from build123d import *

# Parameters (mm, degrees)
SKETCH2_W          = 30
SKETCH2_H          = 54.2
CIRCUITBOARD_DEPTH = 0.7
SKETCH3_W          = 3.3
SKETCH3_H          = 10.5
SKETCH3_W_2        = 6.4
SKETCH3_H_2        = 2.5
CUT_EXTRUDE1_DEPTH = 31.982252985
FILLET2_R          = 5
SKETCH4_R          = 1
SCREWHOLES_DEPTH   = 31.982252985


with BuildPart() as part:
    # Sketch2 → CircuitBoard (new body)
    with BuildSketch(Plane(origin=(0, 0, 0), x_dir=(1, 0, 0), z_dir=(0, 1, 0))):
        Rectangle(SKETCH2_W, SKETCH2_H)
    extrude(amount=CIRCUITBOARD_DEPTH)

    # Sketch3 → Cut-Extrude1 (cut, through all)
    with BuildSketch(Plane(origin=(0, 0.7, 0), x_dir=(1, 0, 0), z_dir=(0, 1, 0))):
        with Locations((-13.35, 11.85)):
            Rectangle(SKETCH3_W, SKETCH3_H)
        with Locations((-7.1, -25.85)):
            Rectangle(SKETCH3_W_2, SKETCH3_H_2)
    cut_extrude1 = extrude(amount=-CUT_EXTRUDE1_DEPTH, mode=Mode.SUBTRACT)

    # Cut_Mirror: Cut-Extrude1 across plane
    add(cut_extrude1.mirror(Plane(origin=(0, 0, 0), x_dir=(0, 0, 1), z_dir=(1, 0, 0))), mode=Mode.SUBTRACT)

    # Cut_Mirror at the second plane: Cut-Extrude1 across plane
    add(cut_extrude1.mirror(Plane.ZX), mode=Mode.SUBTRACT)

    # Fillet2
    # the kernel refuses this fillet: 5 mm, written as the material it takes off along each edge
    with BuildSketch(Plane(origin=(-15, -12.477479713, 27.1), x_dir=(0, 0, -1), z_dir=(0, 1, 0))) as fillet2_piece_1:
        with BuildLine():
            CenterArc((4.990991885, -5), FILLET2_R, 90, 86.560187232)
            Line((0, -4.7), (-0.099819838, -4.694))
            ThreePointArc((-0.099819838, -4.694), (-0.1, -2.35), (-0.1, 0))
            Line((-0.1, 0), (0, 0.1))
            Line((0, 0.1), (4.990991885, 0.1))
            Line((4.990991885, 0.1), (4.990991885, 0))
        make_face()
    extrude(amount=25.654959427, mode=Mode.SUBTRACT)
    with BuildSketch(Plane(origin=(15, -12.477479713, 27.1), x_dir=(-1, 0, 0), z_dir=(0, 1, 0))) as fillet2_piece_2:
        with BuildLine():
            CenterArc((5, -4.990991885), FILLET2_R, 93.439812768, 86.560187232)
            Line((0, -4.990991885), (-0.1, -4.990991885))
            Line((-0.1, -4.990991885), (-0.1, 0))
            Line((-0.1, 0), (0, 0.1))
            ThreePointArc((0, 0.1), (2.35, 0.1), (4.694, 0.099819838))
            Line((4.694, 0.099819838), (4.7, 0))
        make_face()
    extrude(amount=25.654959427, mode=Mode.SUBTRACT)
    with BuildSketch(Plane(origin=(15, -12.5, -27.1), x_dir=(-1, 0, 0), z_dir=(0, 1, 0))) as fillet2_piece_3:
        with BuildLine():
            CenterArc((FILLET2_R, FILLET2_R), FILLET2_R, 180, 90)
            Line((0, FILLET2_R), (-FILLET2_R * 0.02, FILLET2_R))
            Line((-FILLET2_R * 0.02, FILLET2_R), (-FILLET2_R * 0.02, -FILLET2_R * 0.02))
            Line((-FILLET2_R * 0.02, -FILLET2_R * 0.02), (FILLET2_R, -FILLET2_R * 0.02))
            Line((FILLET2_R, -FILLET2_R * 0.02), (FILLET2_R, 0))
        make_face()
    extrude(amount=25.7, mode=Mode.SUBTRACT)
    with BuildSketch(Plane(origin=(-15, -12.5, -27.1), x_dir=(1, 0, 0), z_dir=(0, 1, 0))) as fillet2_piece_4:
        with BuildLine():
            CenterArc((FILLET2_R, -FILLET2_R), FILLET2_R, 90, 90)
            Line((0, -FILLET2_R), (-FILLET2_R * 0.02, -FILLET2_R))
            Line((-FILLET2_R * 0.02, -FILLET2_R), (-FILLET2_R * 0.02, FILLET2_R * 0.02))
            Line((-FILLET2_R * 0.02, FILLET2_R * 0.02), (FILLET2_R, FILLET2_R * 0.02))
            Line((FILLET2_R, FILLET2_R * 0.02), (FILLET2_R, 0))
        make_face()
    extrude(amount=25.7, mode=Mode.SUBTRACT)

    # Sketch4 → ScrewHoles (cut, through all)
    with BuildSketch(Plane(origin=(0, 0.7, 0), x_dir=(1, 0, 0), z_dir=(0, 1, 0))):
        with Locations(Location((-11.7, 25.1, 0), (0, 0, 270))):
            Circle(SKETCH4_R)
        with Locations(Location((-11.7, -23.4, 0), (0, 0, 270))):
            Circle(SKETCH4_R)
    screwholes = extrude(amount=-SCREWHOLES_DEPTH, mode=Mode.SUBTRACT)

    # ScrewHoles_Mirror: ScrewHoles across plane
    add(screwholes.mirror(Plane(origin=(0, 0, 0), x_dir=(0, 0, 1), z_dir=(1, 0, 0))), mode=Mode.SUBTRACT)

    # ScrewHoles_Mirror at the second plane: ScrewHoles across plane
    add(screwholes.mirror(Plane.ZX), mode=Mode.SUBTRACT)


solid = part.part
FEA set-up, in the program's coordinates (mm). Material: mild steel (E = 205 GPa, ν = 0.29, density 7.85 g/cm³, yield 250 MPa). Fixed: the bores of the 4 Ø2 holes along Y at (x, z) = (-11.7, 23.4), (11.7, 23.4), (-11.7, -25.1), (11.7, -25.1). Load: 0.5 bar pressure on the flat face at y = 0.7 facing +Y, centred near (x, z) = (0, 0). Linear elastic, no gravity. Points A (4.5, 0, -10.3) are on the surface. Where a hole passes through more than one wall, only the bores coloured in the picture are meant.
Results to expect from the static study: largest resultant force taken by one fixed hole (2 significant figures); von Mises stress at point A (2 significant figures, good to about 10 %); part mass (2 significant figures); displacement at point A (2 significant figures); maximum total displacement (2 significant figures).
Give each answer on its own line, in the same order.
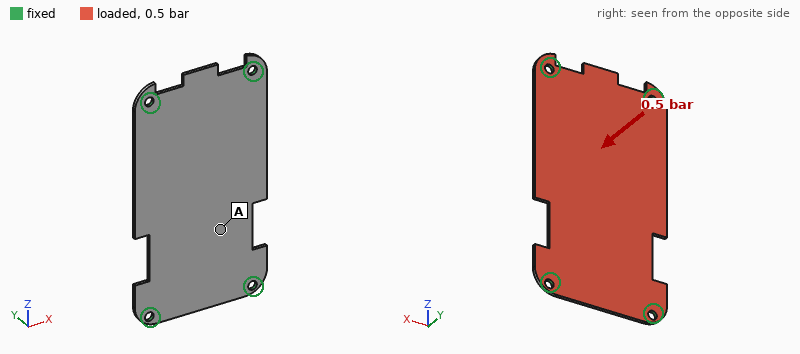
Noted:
19 N
39 MPa
8.2 g
0.11 mm
0.15 mm
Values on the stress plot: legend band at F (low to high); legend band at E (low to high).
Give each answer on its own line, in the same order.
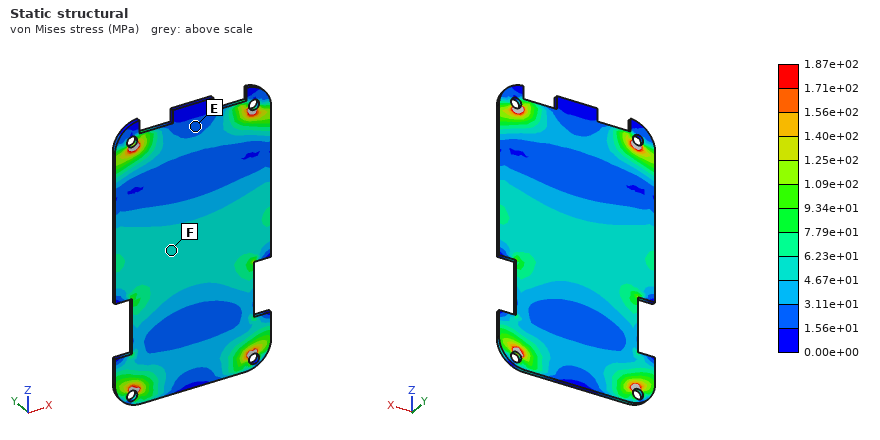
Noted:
4.67e+01 to 6.23e+01 MPa
1.56e+01 to 3.11e+01 MPa
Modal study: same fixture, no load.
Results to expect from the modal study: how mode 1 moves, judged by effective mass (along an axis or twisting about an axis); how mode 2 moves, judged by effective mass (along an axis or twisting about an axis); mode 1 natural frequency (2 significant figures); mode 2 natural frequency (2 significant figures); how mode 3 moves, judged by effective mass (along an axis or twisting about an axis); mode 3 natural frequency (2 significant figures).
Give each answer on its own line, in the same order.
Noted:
along Y
twisting about Z
1400 Hz
2400 Hz
twisting about X
3900 Hz
